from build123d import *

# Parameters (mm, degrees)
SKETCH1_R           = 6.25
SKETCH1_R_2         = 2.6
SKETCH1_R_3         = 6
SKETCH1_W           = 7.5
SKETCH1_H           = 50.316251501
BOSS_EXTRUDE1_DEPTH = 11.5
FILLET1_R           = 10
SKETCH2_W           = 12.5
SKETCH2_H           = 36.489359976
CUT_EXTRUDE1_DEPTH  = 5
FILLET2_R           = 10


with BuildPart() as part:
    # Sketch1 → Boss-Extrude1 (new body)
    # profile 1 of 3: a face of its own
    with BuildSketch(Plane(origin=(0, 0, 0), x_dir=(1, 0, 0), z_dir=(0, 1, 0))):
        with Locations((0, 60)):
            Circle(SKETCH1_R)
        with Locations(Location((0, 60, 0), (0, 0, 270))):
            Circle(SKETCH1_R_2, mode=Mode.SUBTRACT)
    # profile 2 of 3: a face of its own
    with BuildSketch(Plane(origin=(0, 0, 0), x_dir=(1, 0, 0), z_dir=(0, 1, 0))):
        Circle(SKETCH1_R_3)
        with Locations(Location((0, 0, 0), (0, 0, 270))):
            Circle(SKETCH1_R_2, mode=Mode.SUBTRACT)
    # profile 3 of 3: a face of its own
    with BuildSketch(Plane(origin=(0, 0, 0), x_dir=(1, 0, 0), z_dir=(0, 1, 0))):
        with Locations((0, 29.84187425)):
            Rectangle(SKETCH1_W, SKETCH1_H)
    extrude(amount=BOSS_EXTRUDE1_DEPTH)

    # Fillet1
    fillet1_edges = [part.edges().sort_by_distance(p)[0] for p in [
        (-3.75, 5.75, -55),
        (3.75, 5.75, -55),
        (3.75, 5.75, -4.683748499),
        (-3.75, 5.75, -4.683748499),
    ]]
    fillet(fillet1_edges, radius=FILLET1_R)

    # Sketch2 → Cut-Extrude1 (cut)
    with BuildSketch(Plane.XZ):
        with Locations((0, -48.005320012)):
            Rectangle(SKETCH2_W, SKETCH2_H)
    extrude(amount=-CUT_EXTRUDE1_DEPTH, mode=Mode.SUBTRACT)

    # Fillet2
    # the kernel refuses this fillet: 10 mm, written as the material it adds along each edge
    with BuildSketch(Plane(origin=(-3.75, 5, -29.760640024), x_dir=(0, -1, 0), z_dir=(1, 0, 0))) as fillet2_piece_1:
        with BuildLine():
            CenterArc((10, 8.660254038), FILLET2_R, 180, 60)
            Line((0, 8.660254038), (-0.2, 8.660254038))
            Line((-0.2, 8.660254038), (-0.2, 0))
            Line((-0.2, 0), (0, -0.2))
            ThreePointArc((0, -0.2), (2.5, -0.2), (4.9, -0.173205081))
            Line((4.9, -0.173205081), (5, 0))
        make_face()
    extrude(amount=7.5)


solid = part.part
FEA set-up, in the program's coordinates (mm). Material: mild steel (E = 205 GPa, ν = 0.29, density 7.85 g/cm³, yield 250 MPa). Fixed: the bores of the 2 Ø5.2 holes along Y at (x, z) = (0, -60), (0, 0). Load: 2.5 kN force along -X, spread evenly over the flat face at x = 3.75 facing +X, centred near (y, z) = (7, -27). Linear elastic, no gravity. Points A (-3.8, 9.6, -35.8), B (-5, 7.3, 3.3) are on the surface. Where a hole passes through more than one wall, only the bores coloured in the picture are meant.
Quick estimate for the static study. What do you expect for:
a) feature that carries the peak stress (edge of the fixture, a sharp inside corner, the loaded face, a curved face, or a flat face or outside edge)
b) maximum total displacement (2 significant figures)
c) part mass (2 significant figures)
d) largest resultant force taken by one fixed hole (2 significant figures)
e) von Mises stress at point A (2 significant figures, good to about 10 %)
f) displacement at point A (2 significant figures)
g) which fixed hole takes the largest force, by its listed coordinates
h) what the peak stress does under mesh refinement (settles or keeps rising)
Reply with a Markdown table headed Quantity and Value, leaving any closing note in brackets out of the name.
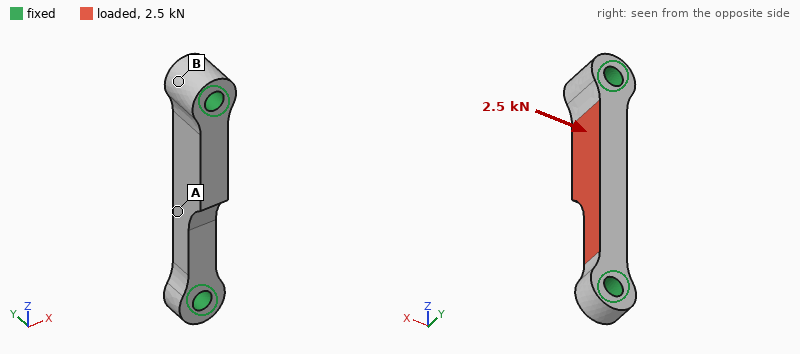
| Quantity | Value |
|---|---|
| feature that carries the peak stress | edge of the fixture |
| maximum total displacement | 28 µm |
| part mass | 40 g |
| largest resultant force taken by one fixed hole | 1.5 kN |
| von Mises stress at point A | 88 MPa |
| displacement at point A | 24 µm |
| which fixed hole takes the largest force, by its listed coordinates | (0, 0) |
| what the peak stress does under mesh refinement | keeps rising |
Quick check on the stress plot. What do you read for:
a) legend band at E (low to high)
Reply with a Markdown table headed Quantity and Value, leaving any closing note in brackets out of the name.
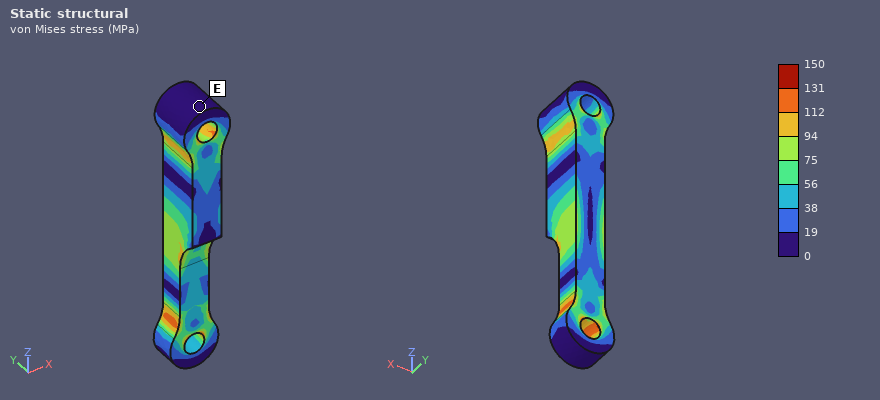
| Quantity | Value |
|---|---|
| legend band at E | 0 to 19 MPa |
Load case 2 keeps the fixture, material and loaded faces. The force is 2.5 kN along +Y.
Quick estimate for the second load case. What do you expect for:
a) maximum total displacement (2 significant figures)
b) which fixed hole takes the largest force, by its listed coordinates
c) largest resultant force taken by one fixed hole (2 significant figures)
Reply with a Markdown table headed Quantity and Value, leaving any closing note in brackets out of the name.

| Quantity | Value |
|---|---|
| maximum total displacement | 29 µm |
| which fixed hole takes the largest force, by its listed coordinates | (0, 0) |
| largest resultant force taken by one fixed hole | 1.6 kN |
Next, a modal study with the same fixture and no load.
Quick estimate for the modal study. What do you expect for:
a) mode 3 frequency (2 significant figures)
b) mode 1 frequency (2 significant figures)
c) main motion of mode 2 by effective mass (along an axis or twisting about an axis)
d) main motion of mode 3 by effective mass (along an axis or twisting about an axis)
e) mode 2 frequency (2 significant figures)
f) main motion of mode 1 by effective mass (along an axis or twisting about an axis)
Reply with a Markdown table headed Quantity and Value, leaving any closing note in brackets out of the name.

| Quantity | Value |
|---|---|
| mode 3 frequency | 24 kHz |
| mode 1 frequency | 11 kHz |
| main motion of mode 2 by effective mass | along Y |
| main motion of mode 3 by effective mass | twisting about Z |
| mode 2 frequency | 12 kHz |
| main motion of mode 1 by effective mass | along X |
